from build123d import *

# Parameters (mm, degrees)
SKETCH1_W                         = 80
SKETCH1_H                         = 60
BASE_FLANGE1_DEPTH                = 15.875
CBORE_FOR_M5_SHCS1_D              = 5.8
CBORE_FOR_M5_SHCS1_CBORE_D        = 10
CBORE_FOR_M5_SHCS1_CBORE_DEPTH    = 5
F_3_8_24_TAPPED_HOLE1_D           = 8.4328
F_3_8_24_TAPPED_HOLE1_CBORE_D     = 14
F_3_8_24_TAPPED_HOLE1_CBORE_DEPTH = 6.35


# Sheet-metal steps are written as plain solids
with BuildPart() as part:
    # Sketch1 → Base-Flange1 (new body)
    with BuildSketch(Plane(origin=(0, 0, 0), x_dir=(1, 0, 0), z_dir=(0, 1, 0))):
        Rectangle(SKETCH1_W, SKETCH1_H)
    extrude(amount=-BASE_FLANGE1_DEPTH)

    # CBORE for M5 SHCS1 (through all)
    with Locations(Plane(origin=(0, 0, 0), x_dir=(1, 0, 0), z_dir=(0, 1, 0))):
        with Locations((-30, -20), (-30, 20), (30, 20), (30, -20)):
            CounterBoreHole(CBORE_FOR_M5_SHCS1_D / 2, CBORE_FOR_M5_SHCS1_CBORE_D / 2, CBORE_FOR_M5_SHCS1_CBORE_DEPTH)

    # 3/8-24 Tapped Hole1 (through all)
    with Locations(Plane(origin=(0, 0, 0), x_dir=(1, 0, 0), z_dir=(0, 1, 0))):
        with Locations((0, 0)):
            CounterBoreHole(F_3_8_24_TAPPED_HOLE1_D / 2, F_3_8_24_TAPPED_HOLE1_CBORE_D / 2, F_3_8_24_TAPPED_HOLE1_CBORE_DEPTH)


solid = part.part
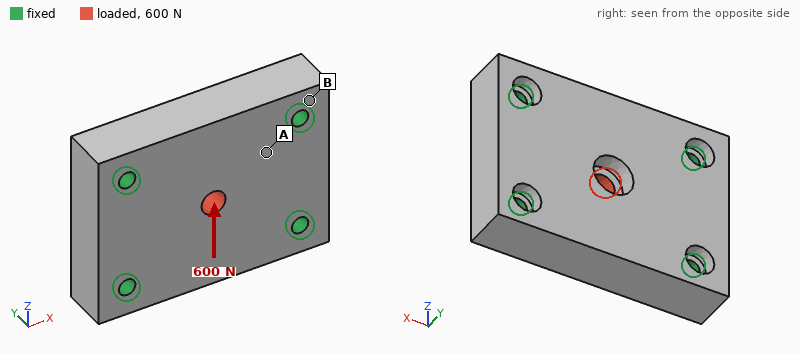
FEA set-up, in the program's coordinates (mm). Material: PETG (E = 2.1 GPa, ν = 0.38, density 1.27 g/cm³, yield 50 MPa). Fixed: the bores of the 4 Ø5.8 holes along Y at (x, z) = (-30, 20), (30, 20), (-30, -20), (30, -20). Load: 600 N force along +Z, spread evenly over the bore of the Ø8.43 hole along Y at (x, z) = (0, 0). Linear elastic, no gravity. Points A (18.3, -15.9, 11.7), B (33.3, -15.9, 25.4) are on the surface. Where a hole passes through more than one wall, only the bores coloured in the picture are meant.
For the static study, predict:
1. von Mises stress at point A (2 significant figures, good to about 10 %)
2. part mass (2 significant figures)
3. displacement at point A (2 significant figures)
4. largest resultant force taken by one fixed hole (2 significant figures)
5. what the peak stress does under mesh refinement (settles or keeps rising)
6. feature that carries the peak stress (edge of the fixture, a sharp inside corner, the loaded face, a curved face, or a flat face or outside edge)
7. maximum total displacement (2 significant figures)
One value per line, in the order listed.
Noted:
1.0 MPa
91 g
8.2 µm
170 N
keeps rising
a sharp inside corner
26 µm
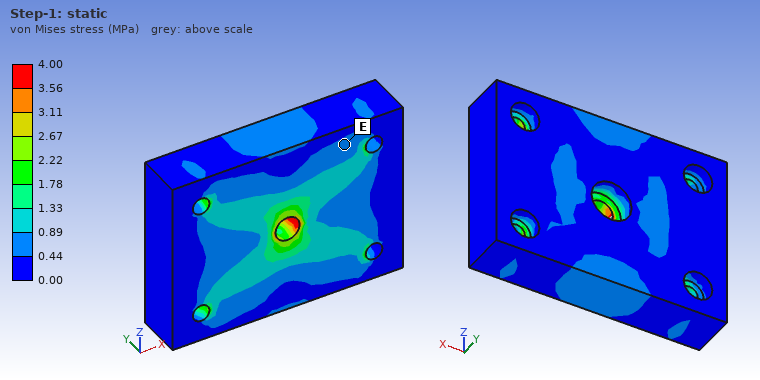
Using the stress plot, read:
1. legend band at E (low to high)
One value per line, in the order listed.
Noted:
0.44 to 0.89 MPa
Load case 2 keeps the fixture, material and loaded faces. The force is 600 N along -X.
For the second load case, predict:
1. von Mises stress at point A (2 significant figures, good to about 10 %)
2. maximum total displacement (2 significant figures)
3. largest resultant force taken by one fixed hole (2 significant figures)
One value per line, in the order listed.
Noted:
0.87 MPa
19 µm
160 N
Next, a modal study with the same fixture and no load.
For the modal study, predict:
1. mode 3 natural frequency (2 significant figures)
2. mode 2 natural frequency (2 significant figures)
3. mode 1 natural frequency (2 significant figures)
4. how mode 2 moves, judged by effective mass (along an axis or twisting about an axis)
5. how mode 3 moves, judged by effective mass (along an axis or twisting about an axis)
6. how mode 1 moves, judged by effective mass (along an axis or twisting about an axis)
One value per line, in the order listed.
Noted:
5300 Hz
4100 Hz
3200 Hz
twisting about X
along Z
along Y
